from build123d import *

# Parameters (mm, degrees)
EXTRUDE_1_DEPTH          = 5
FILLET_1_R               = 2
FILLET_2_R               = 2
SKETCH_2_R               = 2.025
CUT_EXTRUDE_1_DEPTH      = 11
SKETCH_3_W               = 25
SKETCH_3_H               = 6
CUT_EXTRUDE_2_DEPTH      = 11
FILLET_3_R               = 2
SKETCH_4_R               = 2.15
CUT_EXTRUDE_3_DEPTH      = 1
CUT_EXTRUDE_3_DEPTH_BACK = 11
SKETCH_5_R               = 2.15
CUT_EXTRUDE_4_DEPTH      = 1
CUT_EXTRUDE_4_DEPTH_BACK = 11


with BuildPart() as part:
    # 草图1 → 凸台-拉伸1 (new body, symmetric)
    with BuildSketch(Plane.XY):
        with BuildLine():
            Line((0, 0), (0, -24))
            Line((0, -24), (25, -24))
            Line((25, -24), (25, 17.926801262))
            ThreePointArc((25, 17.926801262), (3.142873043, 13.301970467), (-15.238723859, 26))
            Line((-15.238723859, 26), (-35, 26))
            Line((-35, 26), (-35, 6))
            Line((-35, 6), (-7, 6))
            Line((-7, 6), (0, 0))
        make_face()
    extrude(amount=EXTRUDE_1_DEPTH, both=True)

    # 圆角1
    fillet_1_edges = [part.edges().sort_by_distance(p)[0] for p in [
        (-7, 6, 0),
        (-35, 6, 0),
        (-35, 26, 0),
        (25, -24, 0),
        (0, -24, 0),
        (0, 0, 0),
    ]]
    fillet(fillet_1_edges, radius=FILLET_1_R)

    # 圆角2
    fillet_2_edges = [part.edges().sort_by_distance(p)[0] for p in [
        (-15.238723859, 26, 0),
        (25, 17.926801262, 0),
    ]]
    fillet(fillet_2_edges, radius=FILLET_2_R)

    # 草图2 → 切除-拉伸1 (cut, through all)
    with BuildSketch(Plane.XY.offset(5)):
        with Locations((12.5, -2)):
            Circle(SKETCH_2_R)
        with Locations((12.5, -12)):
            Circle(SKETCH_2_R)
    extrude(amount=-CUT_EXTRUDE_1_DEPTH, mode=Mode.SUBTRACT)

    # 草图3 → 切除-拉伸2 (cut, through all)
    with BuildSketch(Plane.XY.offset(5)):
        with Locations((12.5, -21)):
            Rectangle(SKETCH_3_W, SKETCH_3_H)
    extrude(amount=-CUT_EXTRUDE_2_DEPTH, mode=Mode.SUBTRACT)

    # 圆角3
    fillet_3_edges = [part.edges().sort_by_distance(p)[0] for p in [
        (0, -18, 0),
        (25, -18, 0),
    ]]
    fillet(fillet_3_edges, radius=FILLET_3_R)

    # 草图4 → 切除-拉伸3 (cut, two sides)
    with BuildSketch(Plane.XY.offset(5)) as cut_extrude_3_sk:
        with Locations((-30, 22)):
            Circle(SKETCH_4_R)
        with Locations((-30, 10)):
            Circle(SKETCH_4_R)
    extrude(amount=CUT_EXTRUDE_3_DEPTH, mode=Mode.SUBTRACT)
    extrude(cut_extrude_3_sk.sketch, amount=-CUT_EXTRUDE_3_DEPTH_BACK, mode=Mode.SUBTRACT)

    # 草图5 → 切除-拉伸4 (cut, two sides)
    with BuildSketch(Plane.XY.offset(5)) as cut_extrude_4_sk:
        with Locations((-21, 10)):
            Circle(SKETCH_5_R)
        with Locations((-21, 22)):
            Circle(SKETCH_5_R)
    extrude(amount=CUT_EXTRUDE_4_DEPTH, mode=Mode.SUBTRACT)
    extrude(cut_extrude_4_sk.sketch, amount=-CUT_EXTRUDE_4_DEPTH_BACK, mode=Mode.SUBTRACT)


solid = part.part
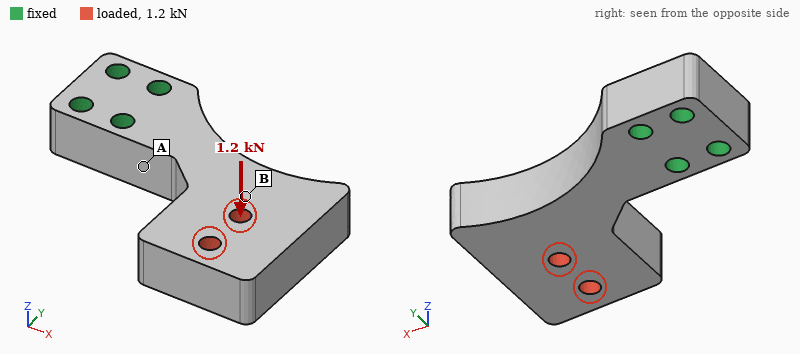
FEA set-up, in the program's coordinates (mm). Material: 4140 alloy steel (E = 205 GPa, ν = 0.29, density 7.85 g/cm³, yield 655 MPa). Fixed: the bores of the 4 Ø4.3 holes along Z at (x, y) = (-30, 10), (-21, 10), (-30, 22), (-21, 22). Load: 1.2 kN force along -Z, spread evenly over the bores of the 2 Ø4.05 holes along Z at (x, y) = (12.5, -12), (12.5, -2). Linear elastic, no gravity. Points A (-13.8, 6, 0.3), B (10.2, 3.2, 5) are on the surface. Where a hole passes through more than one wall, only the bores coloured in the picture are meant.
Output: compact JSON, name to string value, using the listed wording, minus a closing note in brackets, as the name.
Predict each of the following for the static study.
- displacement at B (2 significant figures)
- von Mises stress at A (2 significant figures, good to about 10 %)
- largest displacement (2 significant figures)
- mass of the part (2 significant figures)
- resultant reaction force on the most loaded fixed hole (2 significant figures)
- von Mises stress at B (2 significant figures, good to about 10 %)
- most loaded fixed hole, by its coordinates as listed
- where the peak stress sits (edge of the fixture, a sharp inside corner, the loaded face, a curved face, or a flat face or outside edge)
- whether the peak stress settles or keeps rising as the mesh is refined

{"displacement at B": "0.077 mm", "von Mises stress at A": "120 MPa", "largest displacement": "0.18 mm", "mass of the part": "100 g", "resultant reaction force on the most loaded fixed hole": "2.1 kN", "von Mises stress at B": "30 MPa", "most loaded fixed hole, by its coordinates as listed": "(-21, 10)", "where the peak stress sits": "edge of the fixture", "whether the peak stress settles or keeps rising as the mesh is refined": "keeps rising"}
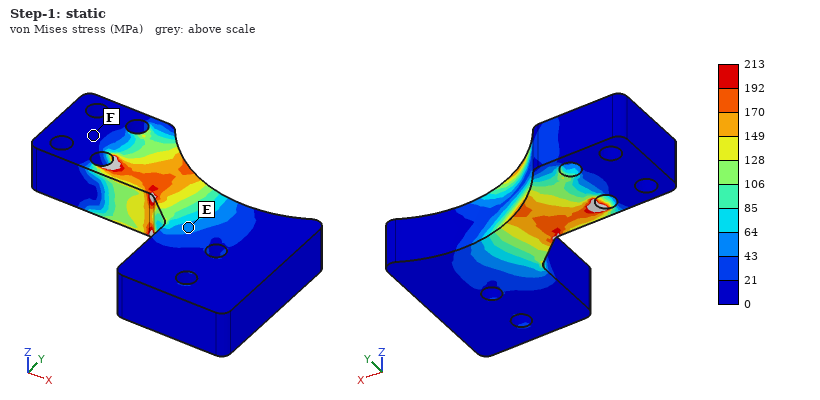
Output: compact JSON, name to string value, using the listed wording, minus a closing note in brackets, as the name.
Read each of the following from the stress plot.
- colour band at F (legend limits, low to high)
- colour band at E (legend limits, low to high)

{"colour band at F": "0 to 21 MPa", "colour band at E": "43 to 64 MPa"}
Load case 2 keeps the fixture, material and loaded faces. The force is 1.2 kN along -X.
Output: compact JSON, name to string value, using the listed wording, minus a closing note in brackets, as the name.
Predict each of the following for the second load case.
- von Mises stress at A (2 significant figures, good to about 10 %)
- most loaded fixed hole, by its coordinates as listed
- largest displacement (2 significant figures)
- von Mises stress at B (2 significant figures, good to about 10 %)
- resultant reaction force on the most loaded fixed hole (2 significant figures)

{"von Mises stress at A": "76 MPa", "most loaded fixed hole, by its coordinates as listed": "(-21, 10)", "largest displacement": "72 µm", "von Mises stress at B": "16 MPa", "resultant reaction force on the most loaded fixed hole": "2.6 kN"}
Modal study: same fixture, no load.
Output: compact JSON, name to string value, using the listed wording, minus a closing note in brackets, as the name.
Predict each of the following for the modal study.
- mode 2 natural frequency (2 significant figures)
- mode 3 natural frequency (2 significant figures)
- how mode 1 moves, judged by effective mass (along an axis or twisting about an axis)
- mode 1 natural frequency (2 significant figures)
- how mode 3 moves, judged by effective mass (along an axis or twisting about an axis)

{"mode 2 natural frequency": "2800 Hz", "mode 3 natural frequency": "5400 Hz", "how mode 1 moves, judged by effective mass": "along Z", "mode 1 natural frequency": "2300 Hz", "how mode 3 moves, judged by effective mass": "twisting about X"}
